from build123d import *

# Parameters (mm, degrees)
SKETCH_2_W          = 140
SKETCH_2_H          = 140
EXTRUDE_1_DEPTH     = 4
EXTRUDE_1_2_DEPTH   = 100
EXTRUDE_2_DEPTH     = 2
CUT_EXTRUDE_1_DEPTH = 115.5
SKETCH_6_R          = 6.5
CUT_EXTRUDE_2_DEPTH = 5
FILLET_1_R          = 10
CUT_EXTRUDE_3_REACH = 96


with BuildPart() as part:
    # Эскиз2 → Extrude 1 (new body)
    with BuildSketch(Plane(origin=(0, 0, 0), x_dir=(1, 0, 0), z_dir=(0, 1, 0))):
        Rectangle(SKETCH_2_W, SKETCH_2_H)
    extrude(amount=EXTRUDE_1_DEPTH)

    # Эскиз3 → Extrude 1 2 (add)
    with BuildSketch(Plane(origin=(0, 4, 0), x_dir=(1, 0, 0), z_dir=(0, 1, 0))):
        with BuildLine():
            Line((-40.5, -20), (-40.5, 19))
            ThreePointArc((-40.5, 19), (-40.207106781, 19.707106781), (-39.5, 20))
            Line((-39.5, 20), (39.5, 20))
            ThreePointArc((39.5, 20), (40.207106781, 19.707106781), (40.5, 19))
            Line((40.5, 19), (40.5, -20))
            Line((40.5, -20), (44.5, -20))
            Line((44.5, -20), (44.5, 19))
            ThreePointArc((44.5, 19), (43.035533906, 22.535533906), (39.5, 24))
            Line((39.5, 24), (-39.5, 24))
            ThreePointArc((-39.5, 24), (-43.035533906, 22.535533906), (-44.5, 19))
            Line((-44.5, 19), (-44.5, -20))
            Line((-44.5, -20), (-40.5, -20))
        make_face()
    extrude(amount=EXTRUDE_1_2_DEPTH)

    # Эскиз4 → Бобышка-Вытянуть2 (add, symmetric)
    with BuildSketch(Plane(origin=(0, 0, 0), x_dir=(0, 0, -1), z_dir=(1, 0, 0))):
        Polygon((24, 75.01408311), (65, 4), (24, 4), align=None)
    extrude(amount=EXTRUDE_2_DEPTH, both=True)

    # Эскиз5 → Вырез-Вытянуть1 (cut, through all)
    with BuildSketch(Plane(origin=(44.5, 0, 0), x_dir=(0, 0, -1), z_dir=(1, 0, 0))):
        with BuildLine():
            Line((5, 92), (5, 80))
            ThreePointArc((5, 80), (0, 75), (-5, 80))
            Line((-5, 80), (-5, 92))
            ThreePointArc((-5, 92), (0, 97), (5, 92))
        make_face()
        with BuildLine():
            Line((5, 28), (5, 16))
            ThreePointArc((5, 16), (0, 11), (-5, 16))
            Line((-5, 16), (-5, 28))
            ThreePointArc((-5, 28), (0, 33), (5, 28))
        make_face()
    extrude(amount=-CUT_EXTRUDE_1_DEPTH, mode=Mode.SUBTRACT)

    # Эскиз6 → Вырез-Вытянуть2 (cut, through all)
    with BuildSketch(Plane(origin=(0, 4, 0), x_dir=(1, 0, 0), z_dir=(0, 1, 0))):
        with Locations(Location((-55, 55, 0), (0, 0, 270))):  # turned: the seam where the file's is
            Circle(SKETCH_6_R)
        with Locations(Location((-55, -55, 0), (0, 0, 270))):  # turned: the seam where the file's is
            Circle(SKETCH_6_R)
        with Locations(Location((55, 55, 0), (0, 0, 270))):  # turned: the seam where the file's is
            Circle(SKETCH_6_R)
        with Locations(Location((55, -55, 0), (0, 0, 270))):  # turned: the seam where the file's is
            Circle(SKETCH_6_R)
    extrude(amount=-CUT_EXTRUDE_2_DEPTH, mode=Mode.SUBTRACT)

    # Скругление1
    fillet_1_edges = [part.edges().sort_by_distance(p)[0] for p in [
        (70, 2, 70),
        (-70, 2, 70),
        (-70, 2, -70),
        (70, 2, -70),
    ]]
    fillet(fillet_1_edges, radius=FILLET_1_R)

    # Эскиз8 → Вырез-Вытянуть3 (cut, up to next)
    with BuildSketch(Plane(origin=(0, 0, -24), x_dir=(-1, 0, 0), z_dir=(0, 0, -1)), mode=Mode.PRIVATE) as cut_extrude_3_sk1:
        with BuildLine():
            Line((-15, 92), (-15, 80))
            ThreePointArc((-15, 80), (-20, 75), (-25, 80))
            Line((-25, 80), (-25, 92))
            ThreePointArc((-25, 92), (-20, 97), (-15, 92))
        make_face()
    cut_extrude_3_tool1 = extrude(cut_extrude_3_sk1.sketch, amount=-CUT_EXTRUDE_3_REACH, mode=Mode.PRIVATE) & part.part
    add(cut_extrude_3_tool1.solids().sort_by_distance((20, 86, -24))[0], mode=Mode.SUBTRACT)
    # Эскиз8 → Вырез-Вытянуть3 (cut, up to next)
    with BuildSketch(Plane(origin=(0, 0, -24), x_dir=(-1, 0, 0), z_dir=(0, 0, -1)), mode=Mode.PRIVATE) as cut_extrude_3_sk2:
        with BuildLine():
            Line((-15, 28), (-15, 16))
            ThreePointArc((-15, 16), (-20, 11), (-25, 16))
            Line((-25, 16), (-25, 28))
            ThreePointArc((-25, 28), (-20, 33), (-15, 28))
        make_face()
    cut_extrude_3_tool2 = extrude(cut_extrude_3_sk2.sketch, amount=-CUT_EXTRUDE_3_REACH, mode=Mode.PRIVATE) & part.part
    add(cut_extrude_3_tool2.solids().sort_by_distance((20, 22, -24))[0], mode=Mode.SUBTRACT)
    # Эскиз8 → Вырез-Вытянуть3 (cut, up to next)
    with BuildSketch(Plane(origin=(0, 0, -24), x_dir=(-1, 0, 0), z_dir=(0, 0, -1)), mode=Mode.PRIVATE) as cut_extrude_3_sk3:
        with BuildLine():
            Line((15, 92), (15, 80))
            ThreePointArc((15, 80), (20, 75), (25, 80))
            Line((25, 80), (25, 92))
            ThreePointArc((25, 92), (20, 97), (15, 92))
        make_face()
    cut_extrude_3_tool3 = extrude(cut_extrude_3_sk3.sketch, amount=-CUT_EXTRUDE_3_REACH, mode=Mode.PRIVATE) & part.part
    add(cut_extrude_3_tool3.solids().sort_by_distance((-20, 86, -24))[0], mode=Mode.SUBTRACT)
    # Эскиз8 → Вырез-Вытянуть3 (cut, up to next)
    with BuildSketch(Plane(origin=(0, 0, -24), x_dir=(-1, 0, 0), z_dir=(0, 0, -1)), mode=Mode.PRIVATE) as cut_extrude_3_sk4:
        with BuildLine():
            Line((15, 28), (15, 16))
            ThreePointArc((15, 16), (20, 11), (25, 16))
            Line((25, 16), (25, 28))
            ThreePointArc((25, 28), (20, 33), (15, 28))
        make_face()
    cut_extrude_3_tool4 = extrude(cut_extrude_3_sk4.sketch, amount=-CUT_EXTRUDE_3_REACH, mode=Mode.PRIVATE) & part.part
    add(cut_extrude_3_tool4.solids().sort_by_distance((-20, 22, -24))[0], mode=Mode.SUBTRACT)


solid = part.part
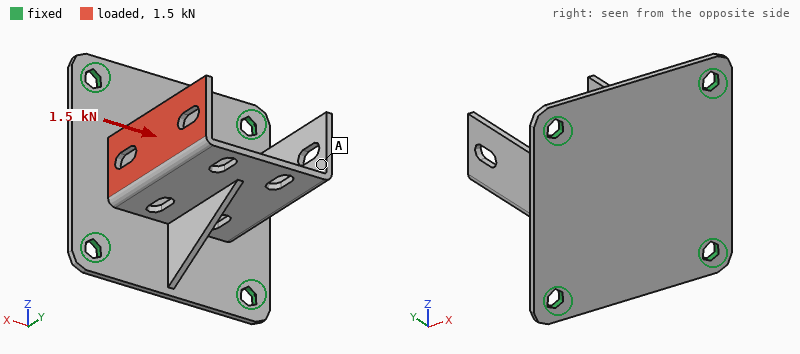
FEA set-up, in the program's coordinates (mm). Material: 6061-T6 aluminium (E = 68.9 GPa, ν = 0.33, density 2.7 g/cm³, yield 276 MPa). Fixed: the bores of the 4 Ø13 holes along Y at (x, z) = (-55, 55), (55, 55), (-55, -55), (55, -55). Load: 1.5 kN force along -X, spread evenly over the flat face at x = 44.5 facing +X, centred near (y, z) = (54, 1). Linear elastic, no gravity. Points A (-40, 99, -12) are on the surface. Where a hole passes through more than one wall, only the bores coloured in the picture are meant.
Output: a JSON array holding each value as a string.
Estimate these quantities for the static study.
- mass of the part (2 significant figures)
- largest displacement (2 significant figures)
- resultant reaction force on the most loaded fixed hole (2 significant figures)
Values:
["380 g", "1.4 mm", "870 N"]
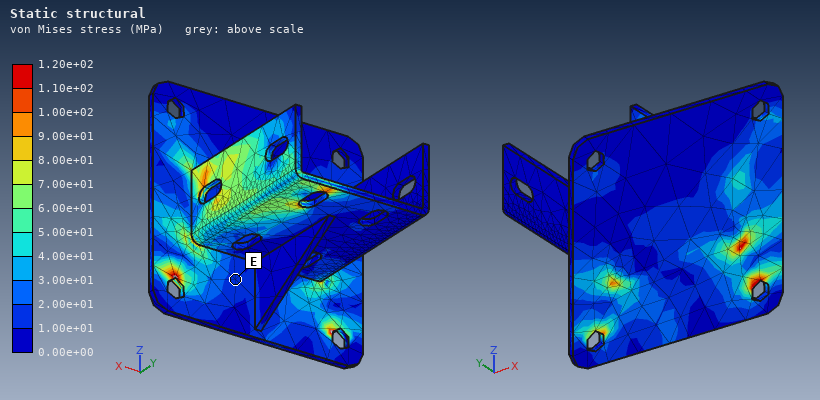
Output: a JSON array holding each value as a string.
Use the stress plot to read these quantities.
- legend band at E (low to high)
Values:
["1.00e+01 to 2.00e+01 MPa"]
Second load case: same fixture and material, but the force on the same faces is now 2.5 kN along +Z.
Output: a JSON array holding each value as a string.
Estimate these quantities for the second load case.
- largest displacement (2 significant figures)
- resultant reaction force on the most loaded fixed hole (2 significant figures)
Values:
["1.4 mm", "1.7 kN"]
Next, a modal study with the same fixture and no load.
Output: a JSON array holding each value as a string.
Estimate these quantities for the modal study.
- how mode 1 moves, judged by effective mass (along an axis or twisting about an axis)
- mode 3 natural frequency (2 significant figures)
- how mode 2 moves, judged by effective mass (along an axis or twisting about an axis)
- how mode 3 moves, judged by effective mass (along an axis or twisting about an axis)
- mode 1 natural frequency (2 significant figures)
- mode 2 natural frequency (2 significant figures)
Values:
["along X", "1200 Hz", "along Z", "along Y", "820 Hz", "930 Hz"]
